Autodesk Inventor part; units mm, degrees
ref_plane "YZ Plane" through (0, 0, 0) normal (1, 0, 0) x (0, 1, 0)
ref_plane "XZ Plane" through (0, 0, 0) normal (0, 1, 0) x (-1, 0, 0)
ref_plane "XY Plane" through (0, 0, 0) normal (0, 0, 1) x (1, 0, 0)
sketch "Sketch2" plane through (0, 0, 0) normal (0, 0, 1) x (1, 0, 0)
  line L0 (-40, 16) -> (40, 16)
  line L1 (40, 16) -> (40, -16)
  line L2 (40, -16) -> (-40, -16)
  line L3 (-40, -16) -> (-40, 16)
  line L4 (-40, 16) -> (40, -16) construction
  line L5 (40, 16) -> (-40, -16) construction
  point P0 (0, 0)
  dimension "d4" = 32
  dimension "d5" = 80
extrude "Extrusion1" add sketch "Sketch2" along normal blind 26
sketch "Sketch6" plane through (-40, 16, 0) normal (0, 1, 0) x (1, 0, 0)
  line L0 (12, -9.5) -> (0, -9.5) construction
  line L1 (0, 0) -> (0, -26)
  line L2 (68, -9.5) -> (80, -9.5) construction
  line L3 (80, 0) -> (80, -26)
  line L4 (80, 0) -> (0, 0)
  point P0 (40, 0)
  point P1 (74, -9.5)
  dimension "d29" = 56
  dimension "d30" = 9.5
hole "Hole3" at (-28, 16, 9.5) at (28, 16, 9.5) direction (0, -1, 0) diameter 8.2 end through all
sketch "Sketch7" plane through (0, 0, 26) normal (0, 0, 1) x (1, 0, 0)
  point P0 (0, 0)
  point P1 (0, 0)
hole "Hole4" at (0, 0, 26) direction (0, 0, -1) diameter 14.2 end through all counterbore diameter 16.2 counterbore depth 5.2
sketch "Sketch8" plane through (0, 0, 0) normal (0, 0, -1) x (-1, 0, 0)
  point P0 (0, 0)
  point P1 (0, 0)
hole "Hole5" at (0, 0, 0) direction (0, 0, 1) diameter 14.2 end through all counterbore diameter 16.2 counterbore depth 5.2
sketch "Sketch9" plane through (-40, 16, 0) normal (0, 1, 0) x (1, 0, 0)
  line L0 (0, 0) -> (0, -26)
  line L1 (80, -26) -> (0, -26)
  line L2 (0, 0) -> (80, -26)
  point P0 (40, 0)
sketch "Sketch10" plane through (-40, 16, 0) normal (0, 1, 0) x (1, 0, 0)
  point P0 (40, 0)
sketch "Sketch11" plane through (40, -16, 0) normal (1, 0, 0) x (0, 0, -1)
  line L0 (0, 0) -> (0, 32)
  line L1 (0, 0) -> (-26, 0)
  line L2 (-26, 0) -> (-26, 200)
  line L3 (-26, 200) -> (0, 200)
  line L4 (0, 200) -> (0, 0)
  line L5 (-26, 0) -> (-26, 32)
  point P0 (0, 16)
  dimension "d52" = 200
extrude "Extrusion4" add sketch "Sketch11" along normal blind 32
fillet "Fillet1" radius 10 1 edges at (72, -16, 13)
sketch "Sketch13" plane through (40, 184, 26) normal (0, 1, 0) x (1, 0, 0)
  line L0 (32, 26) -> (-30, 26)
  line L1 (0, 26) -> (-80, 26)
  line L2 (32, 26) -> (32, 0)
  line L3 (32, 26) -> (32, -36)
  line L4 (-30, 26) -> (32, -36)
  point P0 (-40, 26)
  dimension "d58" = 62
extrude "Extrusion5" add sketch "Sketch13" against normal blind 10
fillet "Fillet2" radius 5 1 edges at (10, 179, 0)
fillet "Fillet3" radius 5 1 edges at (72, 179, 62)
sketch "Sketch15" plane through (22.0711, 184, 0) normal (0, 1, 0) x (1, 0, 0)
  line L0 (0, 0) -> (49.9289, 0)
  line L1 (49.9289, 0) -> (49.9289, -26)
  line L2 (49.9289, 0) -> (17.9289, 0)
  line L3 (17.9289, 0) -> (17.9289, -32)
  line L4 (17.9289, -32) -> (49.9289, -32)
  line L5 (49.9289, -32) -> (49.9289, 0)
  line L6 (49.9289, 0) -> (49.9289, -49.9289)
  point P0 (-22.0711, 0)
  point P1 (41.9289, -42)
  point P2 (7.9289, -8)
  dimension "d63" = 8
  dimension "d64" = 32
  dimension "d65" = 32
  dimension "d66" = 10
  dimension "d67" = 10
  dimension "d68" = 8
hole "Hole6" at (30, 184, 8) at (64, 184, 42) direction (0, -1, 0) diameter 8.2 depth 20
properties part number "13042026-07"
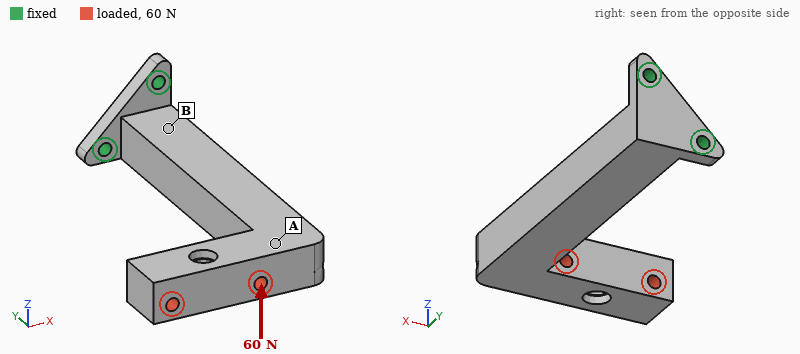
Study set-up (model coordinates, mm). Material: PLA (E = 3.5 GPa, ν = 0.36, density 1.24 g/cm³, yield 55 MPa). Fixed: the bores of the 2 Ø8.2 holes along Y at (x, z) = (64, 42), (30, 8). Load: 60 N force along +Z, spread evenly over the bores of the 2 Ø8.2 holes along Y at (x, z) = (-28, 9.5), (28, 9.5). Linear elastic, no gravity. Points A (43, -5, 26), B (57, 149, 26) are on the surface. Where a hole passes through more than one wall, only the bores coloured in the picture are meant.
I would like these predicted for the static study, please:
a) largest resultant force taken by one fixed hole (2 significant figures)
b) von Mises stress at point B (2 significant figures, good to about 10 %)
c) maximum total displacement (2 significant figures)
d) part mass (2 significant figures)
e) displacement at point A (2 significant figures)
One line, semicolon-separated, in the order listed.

200 N; 2.6 MPa; 2.5 mm; 290 g; 1.9 mm
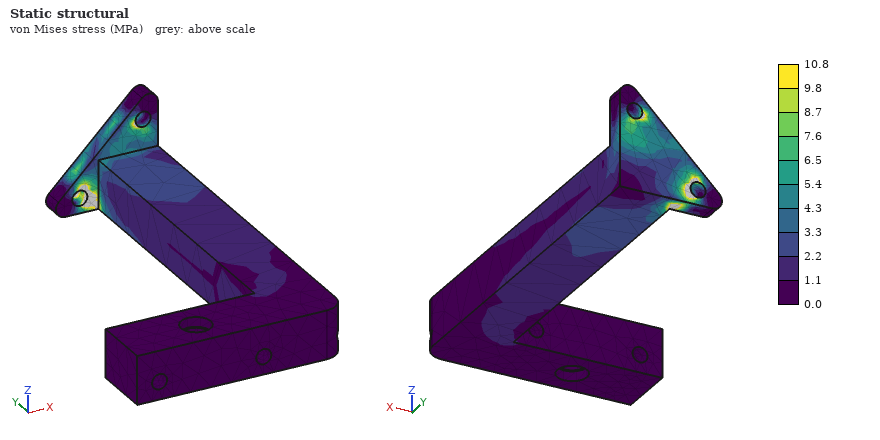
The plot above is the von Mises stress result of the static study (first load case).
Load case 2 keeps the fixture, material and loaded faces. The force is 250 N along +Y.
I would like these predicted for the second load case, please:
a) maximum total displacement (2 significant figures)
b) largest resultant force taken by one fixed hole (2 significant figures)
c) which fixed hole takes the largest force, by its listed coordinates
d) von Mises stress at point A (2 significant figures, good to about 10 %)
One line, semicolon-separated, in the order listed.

2.6 mm; 410 N; (30, 8); 1.3 MPa
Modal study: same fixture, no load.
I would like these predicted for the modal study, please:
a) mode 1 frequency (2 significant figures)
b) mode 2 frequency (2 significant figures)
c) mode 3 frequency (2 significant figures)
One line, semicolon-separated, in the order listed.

67 Hz; 110 Hz; 320 Hz
